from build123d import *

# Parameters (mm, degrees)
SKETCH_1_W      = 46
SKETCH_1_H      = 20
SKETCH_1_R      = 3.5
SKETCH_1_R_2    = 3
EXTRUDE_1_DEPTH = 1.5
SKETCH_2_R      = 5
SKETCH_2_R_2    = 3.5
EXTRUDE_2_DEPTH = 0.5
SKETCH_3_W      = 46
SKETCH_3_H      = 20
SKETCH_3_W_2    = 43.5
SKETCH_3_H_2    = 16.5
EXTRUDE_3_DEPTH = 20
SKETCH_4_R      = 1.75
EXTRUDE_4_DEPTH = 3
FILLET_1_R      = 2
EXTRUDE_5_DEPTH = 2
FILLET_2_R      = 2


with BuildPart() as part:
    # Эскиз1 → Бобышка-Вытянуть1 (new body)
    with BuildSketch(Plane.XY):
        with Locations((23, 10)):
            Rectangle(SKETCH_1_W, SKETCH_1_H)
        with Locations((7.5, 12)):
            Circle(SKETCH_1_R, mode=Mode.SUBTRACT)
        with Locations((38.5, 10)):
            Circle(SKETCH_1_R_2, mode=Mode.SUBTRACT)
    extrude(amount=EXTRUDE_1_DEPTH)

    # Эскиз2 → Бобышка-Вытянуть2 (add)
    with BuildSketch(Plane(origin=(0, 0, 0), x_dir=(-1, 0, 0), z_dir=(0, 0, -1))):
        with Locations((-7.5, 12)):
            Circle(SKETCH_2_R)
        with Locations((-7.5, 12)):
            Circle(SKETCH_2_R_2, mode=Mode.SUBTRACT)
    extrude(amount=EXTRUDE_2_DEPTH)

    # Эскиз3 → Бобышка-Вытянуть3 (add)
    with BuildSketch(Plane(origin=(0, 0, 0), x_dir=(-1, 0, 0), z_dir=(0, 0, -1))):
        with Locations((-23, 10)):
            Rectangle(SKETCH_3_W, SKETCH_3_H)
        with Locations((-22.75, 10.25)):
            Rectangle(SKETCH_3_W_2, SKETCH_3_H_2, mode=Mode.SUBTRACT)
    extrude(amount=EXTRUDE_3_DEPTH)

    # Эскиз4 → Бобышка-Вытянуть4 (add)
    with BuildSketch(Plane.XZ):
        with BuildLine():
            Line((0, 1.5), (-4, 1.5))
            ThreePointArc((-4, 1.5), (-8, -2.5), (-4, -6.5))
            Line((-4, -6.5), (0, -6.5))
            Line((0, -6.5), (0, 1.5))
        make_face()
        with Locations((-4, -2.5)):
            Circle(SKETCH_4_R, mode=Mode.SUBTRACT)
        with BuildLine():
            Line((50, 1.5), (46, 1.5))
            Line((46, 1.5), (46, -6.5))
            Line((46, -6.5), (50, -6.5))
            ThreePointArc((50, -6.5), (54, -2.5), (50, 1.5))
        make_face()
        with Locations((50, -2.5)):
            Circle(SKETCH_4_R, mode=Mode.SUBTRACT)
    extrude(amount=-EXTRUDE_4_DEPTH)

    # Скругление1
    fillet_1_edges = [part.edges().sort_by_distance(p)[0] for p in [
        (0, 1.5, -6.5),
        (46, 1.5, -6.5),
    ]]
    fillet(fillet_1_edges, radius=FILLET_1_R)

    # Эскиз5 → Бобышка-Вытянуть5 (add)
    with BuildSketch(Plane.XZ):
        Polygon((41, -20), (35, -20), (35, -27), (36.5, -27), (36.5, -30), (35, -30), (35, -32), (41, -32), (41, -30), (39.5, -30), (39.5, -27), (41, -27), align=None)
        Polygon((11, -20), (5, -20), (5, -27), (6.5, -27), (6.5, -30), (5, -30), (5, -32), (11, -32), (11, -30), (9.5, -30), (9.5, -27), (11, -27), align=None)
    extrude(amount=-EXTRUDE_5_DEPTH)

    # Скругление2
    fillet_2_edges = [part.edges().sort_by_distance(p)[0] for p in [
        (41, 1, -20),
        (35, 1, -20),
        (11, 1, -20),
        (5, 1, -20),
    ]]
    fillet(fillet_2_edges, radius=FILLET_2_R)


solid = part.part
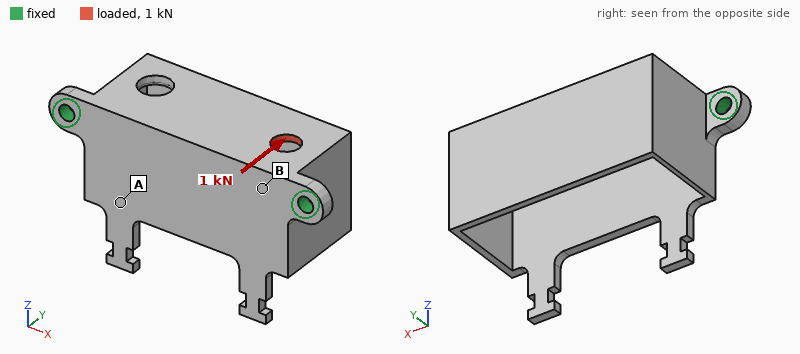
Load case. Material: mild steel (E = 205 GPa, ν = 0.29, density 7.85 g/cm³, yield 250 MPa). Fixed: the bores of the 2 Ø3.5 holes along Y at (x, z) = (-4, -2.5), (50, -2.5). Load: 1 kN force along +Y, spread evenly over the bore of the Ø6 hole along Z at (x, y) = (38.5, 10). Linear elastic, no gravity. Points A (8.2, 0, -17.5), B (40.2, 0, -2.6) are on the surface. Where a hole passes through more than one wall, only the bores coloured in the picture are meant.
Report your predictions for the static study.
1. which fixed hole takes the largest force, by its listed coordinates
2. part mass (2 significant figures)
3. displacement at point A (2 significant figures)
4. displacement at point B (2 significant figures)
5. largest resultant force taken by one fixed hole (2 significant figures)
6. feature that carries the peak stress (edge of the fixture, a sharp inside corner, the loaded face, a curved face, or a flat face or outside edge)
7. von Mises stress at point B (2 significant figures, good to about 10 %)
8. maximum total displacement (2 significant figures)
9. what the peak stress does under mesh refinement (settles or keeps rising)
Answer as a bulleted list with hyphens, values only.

- (50, -2.5)
- 46 g
- 9.2 µm
- 7.2 µm
- 860 N
- edge of the fixture
- 27 MPa
- 41 µm
- keeps rising
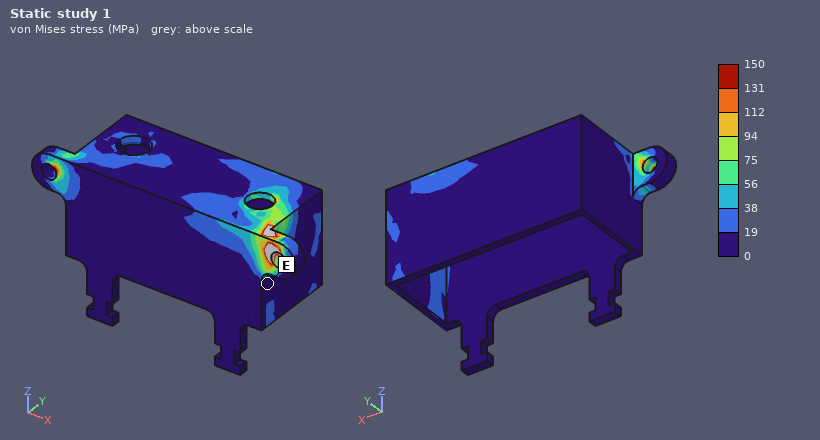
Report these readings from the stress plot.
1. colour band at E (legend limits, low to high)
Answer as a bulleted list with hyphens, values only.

- 0 to 19 MPa
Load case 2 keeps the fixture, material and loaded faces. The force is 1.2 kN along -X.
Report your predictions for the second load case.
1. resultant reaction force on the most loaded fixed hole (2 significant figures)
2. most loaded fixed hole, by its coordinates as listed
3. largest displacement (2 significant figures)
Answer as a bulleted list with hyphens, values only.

- 760 N
- (50, -2.5)
- 12 µm
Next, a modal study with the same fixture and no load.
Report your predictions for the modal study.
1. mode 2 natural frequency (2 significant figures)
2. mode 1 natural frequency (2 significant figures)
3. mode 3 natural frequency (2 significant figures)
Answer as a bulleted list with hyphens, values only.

- 3800 Hz
- 2500 Hz
- 4300 Hz
